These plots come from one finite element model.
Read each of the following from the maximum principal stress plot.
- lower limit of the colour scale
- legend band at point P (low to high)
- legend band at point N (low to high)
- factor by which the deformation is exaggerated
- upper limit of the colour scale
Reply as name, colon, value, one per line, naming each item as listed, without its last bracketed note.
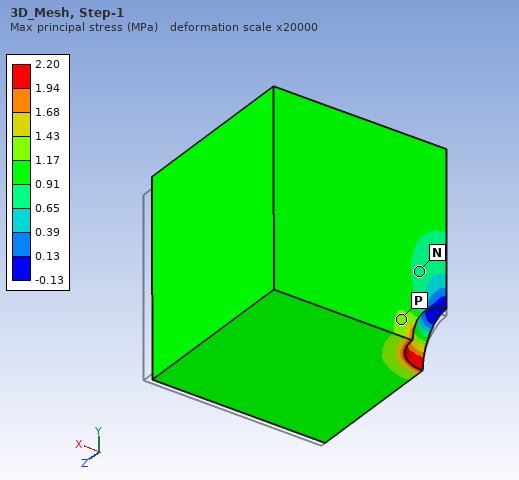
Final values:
lower limit of the colour scale: -0.13 MPa
legend band at point P: 1.17 to 1.43 MPa
legend band at point N: 0.65 to 0.91 MPa
factor by which the deformation is exaggerated: 20000
upper limit of the colour scale: 2.20 MPa
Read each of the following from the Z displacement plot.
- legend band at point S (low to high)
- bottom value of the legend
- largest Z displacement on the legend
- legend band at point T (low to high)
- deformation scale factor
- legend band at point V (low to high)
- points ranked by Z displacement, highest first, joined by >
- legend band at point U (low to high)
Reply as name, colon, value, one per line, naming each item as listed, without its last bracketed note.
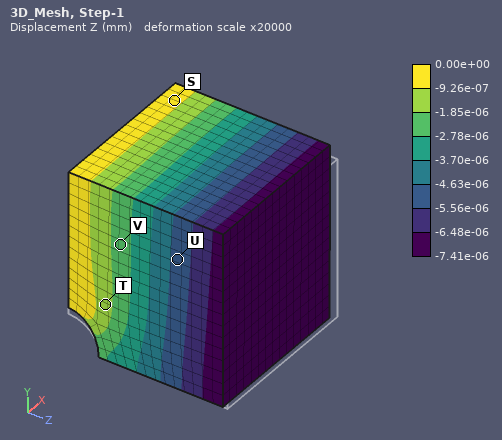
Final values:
legend band at point S: -9.26e-07 to 0.00e+00 mm
bottom value of the legend: -7.41e-06 mm
largest Z displacement on the legend: 0.00e+00 mm
legend band at point T: -1.85e-06 to -9.26e-07 mm
deformation scale factor: 20000
legend band at point V: -2.78e-06 to -1.85e-06 mm
points ranked by Z displacement, highest first, joined by >: S > T > V > U
legend band at point U: -5.56e-06 to -4.63e-06 mm
